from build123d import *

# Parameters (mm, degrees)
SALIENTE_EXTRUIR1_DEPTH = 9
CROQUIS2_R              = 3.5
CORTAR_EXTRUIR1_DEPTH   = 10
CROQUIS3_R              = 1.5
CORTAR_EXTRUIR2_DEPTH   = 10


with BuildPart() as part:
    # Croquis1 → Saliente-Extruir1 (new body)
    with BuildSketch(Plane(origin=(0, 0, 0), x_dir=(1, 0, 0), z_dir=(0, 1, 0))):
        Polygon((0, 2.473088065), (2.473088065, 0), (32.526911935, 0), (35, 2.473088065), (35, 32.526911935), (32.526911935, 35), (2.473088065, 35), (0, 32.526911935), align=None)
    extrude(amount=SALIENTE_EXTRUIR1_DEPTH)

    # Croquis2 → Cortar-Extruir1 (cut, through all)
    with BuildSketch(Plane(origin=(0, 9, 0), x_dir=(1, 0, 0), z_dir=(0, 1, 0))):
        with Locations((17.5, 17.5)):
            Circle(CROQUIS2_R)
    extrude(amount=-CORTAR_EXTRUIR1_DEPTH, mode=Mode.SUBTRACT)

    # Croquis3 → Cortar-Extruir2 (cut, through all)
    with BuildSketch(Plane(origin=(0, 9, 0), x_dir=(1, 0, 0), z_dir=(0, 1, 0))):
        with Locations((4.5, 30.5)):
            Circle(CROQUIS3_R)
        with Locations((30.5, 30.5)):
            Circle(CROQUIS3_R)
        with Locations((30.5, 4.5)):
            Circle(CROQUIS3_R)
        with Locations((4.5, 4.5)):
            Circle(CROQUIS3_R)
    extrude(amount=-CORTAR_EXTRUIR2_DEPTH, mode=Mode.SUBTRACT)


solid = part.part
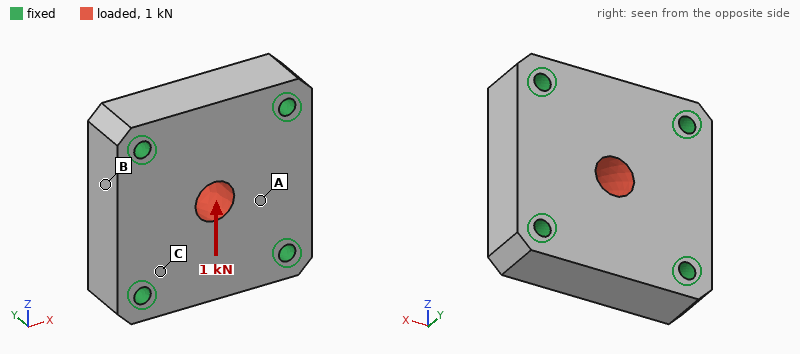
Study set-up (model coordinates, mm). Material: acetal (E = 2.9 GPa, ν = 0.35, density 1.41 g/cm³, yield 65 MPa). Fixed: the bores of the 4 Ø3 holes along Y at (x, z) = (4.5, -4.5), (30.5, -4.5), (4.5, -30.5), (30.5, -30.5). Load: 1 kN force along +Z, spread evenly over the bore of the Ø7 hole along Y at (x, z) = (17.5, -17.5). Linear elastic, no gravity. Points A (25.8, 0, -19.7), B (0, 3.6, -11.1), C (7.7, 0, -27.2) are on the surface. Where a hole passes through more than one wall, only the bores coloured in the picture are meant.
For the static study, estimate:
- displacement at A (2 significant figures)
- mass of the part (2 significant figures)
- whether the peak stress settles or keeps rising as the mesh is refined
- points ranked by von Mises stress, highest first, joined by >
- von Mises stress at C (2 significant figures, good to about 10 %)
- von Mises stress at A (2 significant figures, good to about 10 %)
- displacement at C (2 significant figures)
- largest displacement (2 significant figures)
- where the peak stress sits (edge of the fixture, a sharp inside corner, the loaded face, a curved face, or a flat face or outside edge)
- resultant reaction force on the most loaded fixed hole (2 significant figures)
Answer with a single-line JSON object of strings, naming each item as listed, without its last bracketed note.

{"displacement at A": "11 µm", "mass of the part": "15 g", "whether the peak stress settles or keeps rising as the mesh is refined": "keeps rising", "points ranked by von Mises stress, highest first, joined by >": "C > A > B", "von Mises stress at C": "4.2 MPa", "von Mises stress at A": "2.6 MPa", "displacement at C": "6.7 µm", "largest displacement": "27 µm", "where the peak stress sits": "edge of the fixture", "resultant reaction force on the most loaded fixed hole": "280 N"}
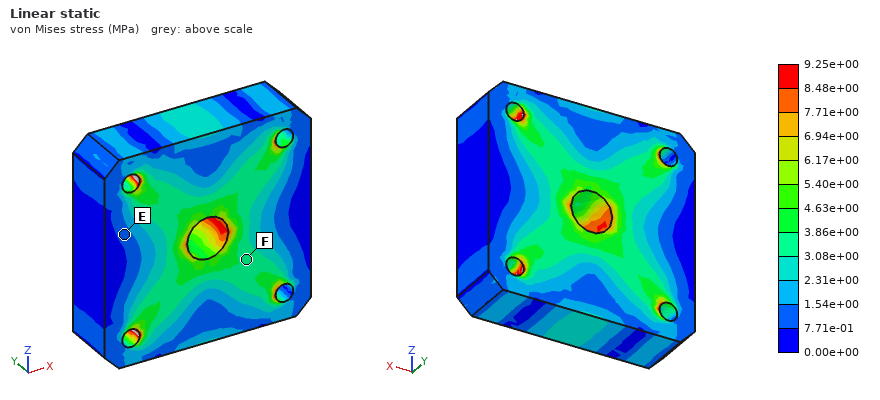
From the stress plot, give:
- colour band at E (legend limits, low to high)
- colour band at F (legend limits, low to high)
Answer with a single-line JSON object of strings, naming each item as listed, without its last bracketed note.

{"colour band at E": "7.71e-01 to 1.54e+00 MPa", "colour band at F": "3.08e+00 to 3.86e+00 MPa"}
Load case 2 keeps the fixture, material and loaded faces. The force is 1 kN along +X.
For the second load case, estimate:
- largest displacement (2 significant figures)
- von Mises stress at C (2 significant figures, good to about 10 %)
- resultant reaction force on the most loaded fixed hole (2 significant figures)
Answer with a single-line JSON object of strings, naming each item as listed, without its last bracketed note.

{"largest displacement": "27 µm", "von Mises stress at C": "4.2 MPa", "resultant reaction force on the most loaded fixed hole": "280 N"}
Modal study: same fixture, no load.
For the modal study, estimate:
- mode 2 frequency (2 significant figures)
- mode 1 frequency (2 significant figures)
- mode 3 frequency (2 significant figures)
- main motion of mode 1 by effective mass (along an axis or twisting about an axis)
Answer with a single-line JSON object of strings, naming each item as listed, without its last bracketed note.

{"mode 2 frequency": "13 kHz", "mode 1 frequency": "9200 Hz", "mode 3 frequency": "13 kHz", "main motion of mode 1 by effective mass": "along Y"}
